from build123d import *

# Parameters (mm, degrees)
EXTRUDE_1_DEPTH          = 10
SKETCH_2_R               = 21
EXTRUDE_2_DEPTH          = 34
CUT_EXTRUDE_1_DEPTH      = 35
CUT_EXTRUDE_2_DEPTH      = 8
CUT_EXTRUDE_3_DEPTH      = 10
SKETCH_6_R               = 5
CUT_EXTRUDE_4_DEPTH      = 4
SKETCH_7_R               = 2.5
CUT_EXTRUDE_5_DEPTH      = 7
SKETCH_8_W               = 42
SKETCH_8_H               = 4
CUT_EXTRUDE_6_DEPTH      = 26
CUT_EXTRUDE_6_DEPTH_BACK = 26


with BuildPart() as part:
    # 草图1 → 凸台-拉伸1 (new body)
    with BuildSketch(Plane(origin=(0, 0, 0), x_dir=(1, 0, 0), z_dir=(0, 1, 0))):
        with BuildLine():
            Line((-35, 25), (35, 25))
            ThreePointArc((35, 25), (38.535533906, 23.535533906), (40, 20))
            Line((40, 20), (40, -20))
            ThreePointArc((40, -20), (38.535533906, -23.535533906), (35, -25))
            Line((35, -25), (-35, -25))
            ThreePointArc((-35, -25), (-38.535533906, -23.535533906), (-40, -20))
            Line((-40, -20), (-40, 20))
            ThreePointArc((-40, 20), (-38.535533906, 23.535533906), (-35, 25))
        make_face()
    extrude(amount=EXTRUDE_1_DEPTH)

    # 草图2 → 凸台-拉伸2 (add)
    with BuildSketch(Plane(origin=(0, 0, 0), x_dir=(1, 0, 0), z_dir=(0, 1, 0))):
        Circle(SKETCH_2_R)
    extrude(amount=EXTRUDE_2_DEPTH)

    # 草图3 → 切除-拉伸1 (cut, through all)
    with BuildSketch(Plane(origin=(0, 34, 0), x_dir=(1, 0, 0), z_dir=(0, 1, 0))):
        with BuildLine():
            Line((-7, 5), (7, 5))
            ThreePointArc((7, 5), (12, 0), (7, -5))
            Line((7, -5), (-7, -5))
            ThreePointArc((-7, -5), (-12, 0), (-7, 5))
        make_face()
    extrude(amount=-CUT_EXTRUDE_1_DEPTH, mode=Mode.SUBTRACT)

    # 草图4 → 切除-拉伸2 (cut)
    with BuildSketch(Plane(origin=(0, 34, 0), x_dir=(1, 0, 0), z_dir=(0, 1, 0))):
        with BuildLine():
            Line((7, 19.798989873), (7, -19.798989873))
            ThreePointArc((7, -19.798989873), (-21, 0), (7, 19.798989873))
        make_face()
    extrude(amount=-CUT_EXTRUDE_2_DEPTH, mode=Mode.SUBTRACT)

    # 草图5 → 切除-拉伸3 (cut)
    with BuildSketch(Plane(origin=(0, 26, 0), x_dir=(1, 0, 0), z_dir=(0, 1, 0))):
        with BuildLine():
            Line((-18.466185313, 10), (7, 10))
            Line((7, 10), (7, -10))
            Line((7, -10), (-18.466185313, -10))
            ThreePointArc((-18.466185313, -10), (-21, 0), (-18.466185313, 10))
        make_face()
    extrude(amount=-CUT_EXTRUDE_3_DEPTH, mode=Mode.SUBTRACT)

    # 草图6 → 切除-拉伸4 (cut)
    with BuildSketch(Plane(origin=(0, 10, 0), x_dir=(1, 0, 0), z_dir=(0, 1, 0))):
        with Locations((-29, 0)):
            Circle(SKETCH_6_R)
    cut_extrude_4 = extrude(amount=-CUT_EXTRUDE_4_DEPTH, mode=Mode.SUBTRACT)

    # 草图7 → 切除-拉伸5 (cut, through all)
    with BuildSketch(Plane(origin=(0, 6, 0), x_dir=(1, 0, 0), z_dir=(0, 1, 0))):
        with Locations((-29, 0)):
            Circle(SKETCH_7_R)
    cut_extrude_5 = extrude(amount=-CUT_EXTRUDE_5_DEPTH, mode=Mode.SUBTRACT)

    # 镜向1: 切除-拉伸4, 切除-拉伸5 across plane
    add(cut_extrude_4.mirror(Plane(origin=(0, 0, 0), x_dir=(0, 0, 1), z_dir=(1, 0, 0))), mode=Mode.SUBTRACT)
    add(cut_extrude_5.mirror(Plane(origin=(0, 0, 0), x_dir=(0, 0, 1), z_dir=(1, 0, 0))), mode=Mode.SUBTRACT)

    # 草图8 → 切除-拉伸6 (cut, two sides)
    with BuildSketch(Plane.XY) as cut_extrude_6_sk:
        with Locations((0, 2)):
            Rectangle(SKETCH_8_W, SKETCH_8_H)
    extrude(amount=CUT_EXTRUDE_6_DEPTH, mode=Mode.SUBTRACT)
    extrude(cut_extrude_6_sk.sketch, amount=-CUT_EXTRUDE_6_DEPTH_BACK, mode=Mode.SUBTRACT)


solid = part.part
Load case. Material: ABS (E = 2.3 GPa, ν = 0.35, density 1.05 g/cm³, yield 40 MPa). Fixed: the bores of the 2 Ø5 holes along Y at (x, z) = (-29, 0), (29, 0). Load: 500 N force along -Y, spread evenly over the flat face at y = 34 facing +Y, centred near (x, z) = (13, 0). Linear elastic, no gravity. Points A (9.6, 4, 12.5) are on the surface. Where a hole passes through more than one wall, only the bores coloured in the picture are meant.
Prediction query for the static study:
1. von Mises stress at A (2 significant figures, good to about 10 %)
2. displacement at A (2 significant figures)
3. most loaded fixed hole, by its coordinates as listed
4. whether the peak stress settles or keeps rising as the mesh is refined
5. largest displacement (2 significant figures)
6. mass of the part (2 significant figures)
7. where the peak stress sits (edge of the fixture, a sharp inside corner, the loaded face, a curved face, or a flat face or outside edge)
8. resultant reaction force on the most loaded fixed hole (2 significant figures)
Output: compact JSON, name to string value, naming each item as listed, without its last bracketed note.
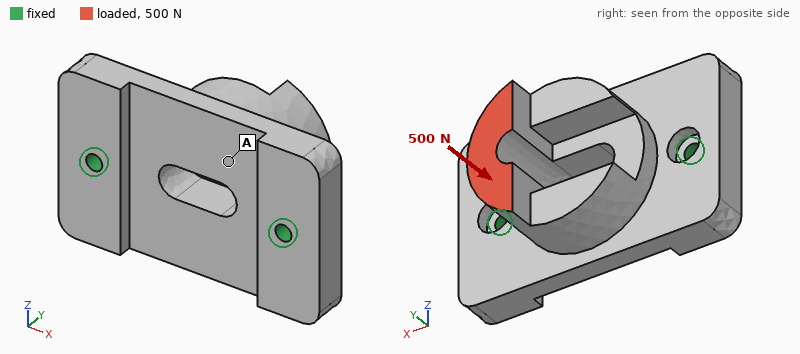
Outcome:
{"von Mises stress at A": "1.4 MPa", "displacement at A": "71 µm", "most loaded fixed hole, by its coordinates as listed": "(29, 0)", "whether the peak stress settles or keeps rising as the mesh is refined": "keeps rising", "largest displacement": "88 µm", "mass of the part": "50 g", "where the peak stress sits": "edge of the fixture", "resultant reaction force on the most loaded fixed hole": "430 N"}
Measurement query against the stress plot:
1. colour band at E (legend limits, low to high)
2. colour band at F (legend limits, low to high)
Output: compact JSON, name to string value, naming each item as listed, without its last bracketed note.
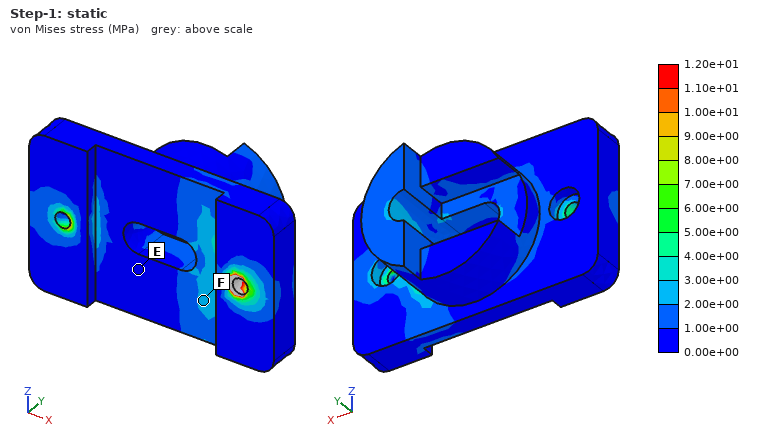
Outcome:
{"colour band at E": "0.00e+00 to 1.00e+00 MPa", "colour band at F": "2.00e+00 to 3.00e+00 MPa"}
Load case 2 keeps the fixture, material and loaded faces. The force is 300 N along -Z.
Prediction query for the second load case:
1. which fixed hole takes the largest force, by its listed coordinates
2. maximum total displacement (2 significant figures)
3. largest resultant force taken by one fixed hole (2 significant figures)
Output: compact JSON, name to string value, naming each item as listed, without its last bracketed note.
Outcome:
{"which fixed hole takes the largest force, by its listed coordinates": "(29, 0)", "maximum total displacement": "0.76 mm", "largest resultant force taken by one fixed hole": "210 N"}
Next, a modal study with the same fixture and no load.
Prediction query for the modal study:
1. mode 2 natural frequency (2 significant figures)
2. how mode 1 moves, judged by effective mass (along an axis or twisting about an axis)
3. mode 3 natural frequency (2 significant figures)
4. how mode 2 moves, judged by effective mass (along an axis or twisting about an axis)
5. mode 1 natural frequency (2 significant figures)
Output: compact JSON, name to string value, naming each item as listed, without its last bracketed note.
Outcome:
{"mode 2 natural frequency": "2400 Hz", "how mode 1 moves, judged by effective mass": "along Z", "mode 3 natural frequency": "2700 Hz", "how mode 2 moves, judged by effective mass": "along Y", "mode 1 natural frequency": "970 Hz"}
